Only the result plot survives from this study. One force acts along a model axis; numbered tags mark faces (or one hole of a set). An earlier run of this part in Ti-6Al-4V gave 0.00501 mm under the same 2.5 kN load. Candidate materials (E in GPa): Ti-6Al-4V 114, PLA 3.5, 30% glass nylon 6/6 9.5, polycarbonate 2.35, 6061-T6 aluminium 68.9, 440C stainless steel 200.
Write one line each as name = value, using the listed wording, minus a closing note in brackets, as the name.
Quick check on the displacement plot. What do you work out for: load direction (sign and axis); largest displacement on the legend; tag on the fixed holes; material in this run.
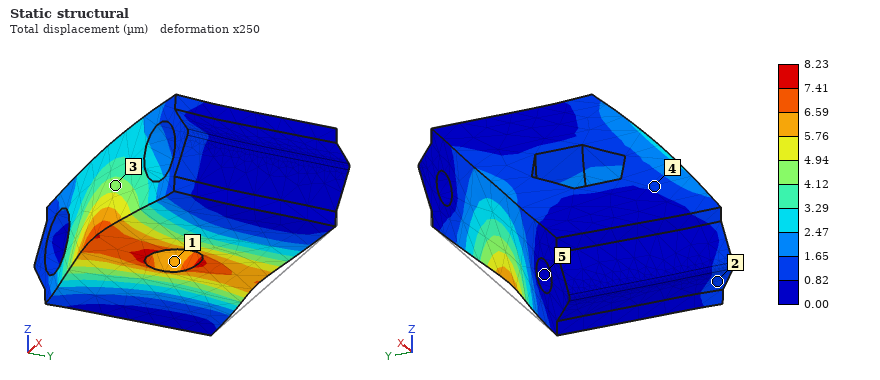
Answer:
load direction = -Y
largest displacement on the legend = 8.23 µm
tag on the fixed holes = 5
material in this run = 6061-T6 aluminium
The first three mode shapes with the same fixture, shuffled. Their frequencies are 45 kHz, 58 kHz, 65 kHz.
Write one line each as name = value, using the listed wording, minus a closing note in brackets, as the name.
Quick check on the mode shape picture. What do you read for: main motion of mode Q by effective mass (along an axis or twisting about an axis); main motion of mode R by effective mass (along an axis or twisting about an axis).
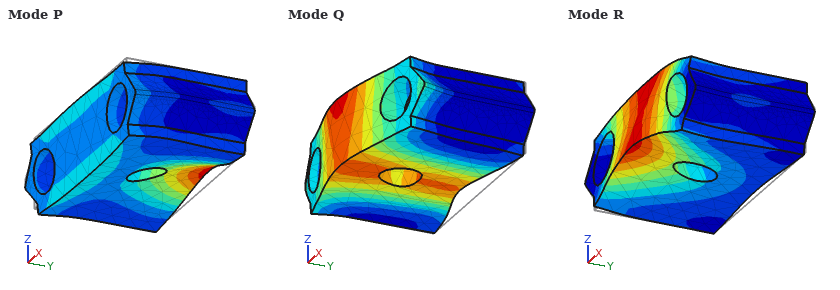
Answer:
main motion of mode Q by effective mass = along Y
main motion of mode R by effective mass = along Z
